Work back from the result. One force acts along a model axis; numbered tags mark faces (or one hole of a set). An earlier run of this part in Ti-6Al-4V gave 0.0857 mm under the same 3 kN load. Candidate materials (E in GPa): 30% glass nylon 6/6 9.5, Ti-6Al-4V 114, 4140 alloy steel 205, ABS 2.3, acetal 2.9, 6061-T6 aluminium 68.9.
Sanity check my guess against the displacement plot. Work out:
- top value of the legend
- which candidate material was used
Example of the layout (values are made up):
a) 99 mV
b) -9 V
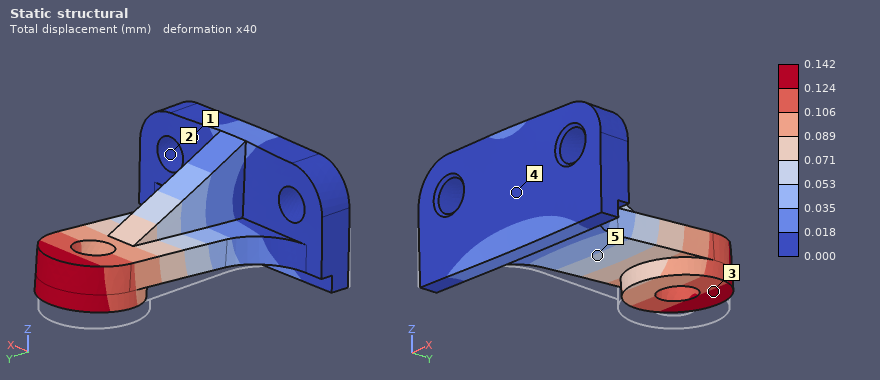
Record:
a) 0.142 mm
b) 6061-T6 aluminium
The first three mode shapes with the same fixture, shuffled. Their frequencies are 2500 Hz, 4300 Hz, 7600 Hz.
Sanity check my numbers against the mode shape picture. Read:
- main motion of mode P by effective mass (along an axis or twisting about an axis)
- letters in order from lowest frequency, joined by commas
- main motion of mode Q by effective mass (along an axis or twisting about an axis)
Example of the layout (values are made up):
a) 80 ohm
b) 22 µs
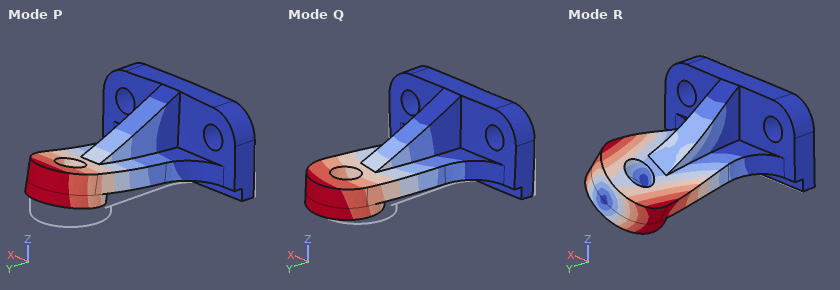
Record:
a) along Z
b) P, Q, R
c) along X
